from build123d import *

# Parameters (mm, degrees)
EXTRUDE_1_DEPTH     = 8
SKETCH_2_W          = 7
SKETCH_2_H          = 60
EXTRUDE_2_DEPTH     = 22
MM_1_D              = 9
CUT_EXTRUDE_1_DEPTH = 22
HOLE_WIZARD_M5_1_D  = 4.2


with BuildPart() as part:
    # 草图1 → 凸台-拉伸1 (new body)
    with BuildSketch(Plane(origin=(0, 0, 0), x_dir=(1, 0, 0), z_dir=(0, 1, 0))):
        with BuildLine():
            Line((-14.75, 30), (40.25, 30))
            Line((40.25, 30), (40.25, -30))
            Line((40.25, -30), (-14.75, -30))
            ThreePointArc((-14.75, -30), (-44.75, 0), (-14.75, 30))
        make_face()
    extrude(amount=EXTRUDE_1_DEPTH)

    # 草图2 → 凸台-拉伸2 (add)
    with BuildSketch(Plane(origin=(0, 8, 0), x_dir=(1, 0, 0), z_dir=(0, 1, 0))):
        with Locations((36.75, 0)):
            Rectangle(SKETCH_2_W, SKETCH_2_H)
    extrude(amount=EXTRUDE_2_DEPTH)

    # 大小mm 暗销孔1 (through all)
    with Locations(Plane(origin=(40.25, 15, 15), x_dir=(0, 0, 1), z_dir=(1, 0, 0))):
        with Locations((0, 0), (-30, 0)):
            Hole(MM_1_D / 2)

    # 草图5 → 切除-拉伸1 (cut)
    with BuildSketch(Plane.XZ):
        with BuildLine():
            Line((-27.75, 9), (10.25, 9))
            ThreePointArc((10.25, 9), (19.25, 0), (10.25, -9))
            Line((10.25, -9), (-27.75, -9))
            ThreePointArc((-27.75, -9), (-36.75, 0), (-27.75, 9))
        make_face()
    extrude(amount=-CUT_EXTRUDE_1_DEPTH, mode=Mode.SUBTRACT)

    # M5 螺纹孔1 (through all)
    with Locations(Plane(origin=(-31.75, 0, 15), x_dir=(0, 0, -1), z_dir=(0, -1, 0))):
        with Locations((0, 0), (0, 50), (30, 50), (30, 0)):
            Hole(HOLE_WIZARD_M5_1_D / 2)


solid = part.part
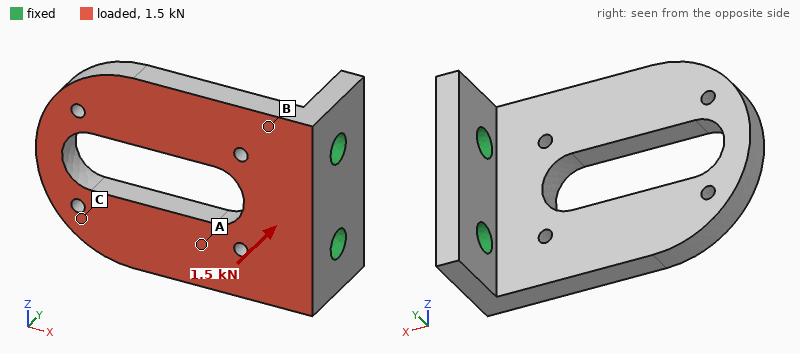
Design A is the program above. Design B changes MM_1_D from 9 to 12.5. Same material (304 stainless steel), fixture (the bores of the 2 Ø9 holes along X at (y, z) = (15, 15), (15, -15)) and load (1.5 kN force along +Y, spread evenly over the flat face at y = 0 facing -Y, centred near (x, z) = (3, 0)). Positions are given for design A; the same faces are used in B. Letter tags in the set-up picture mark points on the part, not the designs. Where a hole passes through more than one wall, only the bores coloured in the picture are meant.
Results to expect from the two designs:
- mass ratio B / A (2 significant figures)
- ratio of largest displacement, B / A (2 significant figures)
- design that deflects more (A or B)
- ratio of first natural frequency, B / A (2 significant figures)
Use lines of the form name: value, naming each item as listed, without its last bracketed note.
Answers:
mass ratio B / A: 0.98
ratio of largest displacement, B / A: 0.90
design that deflects more: A
ratio of first natural frequency, B / A: 1.1
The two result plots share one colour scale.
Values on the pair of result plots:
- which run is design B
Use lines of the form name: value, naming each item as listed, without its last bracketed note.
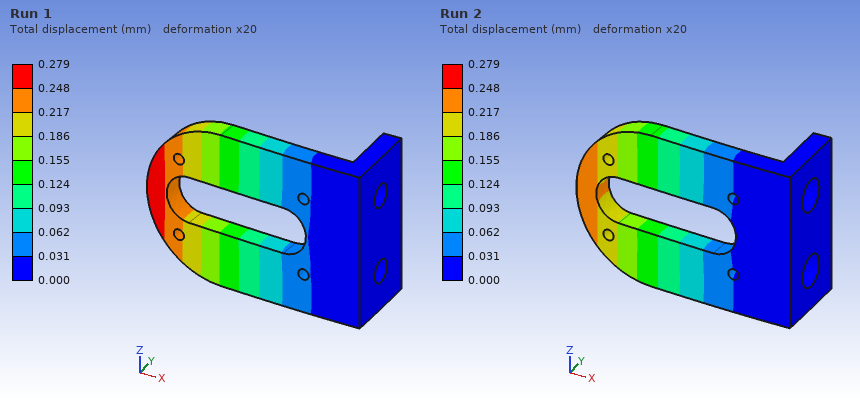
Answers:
which run is design B: Run 2
